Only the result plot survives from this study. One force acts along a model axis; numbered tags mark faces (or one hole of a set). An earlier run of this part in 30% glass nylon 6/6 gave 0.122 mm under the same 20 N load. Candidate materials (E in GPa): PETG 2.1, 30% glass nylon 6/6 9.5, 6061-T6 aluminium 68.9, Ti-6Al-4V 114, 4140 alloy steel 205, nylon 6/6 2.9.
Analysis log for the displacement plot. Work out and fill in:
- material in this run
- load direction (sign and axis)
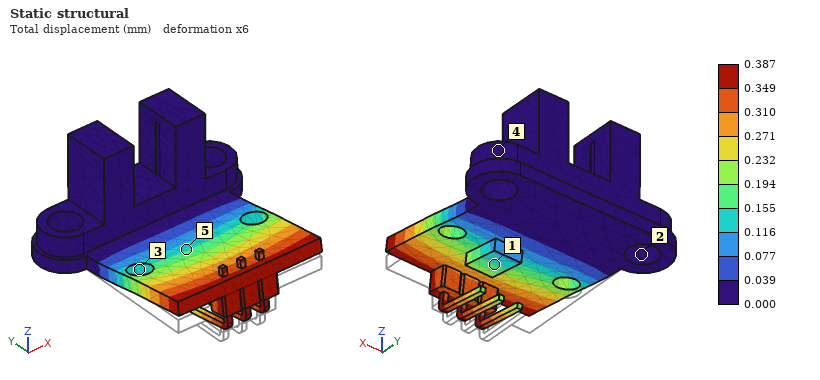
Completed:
nylon 6/6
+Z
